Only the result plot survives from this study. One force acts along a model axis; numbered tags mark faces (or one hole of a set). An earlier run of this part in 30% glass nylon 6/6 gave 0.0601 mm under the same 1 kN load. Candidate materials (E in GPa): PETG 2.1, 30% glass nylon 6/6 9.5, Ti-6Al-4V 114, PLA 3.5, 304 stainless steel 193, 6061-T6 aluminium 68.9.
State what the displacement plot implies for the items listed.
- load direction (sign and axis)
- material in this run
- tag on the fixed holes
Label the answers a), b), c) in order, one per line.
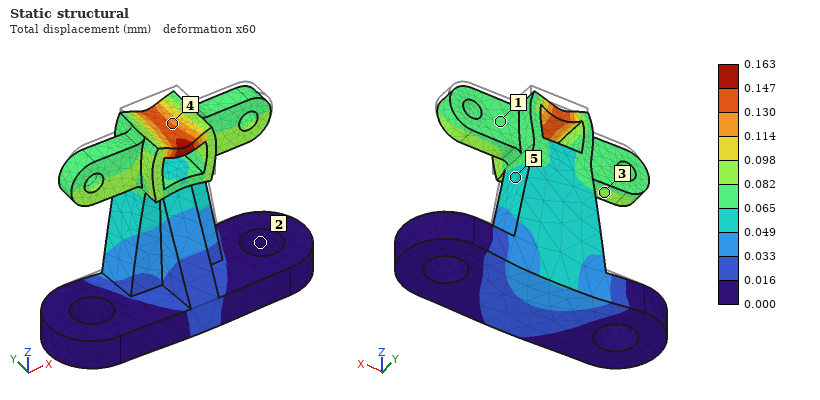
a) -Z
b) PLA
c) 2
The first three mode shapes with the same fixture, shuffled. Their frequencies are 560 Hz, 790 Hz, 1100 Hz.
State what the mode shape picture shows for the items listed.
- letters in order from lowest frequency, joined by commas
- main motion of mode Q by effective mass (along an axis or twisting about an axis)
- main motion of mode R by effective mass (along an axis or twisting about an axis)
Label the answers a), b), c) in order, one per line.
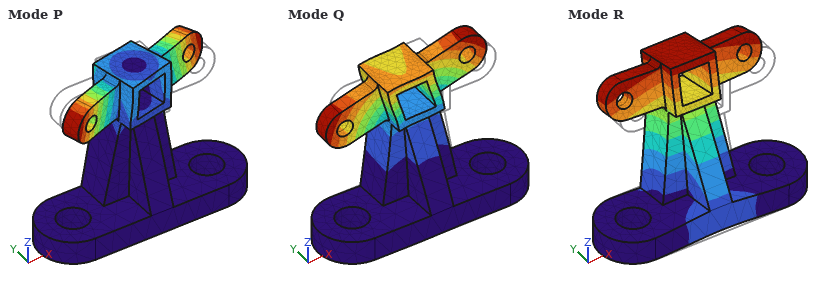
a) R, Q, P
b) along X
c) along Y
